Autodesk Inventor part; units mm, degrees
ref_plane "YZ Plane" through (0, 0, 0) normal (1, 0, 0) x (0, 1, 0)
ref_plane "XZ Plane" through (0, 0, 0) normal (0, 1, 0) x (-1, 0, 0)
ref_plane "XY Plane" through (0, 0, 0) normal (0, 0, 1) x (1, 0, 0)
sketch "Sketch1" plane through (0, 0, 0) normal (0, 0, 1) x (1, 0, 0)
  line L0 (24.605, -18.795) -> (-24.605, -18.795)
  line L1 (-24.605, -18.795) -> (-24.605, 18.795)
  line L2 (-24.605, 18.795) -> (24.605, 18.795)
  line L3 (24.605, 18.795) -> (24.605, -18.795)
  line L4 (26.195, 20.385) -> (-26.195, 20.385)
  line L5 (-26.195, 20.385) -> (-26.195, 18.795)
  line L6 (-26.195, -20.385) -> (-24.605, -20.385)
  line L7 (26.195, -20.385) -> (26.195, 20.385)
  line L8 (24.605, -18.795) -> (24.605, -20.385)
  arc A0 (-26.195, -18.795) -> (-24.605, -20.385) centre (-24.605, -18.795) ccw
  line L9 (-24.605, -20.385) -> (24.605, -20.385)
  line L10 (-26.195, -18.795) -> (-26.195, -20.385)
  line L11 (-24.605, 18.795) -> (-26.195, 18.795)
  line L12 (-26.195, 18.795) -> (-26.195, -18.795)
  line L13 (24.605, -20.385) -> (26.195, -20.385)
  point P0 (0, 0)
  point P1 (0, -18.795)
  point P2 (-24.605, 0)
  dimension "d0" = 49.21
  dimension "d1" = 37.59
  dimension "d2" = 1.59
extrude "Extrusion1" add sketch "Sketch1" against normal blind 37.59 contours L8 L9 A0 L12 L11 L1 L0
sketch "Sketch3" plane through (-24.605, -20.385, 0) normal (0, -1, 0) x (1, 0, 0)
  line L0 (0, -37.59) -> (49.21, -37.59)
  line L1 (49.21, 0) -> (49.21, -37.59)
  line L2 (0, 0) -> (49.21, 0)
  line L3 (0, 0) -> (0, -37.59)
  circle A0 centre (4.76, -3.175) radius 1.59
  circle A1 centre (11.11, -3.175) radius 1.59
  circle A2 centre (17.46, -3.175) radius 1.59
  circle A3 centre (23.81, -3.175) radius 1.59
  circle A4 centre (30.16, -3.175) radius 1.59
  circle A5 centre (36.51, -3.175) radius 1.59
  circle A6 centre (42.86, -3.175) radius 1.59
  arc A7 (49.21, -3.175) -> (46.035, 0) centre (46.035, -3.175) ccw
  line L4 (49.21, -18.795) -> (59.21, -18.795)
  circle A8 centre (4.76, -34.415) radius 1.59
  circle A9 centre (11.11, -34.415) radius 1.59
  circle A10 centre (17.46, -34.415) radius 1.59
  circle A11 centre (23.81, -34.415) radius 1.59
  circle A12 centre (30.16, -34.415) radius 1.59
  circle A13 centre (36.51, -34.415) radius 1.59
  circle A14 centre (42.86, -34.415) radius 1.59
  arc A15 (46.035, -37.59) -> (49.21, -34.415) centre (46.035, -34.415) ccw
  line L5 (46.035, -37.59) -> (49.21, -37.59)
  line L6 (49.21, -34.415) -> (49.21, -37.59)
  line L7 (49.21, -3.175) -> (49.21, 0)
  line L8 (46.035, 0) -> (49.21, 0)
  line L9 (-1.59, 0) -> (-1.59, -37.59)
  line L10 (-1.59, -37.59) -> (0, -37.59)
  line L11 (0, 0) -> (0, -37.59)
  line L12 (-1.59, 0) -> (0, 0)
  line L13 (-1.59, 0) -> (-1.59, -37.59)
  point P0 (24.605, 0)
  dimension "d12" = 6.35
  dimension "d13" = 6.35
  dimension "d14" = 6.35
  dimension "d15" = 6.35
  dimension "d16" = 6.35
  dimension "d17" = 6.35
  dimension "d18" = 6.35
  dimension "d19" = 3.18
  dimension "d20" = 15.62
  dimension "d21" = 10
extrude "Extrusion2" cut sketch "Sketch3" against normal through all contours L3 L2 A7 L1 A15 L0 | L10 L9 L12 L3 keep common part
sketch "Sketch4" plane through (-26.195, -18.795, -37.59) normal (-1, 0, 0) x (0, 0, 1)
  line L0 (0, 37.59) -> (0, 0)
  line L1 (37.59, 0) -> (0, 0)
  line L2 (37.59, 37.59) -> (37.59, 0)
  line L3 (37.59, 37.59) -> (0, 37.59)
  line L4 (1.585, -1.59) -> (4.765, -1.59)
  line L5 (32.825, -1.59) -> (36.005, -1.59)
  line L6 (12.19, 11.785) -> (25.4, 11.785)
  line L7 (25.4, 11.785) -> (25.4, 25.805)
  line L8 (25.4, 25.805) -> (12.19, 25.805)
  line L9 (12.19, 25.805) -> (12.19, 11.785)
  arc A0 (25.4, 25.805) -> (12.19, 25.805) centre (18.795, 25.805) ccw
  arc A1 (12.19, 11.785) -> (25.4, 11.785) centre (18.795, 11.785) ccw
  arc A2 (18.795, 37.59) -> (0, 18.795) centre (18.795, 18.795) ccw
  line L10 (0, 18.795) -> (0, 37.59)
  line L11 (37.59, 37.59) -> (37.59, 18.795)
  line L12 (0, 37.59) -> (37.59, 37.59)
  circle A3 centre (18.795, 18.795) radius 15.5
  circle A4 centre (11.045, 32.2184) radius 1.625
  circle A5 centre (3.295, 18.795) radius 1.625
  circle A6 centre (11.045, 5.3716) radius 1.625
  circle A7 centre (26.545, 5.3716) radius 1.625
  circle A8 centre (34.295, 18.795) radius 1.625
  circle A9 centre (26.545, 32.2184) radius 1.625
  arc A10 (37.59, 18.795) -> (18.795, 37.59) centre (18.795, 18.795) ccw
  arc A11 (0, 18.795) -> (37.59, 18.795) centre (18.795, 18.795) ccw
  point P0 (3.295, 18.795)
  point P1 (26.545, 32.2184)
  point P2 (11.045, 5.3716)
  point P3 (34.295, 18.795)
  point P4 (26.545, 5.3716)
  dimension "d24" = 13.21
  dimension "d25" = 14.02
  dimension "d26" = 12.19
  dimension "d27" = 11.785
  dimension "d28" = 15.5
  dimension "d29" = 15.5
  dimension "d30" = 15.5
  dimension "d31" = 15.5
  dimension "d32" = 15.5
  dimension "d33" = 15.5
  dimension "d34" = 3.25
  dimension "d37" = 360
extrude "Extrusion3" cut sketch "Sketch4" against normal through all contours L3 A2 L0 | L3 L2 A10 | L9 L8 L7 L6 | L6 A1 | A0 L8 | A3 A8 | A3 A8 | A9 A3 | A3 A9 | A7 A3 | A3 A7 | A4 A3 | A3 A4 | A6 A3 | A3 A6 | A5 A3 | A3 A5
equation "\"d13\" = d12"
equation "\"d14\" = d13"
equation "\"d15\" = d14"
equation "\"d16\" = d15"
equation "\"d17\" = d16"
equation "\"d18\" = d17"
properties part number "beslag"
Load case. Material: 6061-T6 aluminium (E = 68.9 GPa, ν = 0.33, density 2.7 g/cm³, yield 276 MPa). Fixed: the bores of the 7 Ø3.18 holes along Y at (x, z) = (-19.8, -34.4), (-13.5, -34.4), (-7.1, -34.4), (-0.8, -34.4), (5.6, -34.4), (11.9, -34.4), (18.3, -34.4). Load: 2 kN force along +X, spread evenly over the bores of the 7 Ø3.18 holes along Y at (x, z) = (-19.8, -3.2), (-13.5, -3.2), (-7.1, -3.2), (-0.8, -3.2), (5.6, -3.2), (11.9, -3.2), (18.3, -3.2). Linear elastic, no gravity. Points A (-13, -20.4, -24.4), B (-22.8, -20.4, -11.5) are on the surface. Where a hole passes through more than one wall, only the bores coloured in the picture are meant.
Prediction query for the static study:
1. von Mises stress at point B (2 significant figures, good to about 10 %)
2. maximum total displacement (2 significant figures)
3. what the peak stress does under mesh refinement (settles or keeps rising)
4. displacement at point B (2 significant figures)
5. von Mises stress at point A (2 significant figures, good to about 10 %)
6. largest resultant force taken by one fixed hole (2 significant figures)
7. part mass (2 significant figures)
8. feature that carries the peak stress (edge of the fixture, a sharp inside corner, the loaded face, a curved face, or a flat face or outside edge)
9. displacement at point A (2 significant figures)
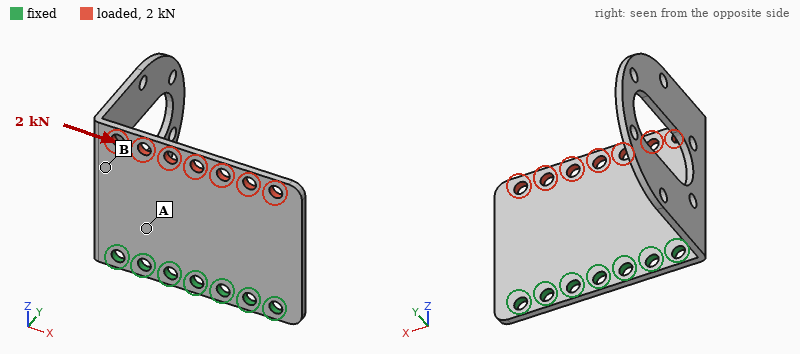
25 MPa
70 µm
keeps rising
44 µm
64 MPa
1.3 kN
11 g
edge of the fixture
15 µm
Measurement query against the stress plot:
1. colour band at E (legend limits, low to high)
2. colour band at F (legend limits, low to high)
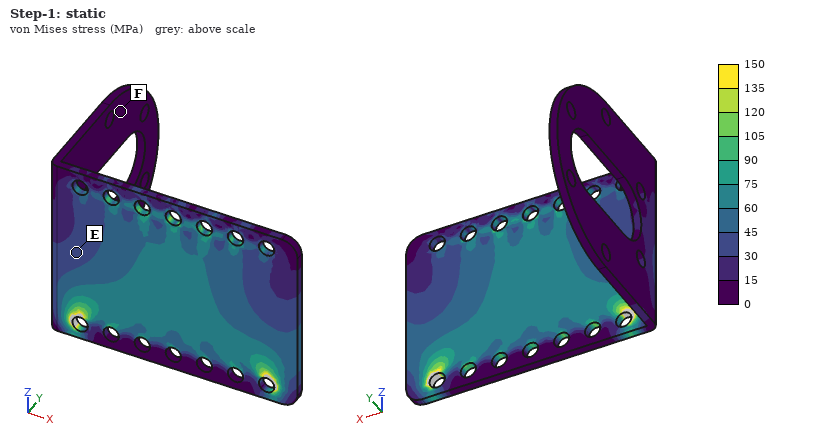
30 to 45 MPa
0 to 15 MPa
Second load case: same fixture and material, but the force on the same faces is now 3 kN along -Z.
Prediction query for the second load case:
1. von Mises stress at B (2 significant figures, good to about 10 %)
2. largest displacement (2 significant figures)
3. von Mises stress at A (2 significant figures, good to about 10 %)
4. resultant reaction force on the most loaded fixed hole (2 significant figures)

24 MPa
21 µm
41 MPa
580 N
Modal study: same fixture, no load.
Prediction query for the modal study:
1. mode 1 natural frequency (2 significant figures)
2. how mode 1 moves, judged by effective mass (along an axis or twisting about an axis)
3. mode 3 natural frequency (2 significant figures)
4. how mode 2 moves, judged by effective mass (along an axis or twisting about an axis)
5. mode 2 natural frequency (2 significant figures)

770 Hz
along X
1700 Hz
along Y
1100 Hz
